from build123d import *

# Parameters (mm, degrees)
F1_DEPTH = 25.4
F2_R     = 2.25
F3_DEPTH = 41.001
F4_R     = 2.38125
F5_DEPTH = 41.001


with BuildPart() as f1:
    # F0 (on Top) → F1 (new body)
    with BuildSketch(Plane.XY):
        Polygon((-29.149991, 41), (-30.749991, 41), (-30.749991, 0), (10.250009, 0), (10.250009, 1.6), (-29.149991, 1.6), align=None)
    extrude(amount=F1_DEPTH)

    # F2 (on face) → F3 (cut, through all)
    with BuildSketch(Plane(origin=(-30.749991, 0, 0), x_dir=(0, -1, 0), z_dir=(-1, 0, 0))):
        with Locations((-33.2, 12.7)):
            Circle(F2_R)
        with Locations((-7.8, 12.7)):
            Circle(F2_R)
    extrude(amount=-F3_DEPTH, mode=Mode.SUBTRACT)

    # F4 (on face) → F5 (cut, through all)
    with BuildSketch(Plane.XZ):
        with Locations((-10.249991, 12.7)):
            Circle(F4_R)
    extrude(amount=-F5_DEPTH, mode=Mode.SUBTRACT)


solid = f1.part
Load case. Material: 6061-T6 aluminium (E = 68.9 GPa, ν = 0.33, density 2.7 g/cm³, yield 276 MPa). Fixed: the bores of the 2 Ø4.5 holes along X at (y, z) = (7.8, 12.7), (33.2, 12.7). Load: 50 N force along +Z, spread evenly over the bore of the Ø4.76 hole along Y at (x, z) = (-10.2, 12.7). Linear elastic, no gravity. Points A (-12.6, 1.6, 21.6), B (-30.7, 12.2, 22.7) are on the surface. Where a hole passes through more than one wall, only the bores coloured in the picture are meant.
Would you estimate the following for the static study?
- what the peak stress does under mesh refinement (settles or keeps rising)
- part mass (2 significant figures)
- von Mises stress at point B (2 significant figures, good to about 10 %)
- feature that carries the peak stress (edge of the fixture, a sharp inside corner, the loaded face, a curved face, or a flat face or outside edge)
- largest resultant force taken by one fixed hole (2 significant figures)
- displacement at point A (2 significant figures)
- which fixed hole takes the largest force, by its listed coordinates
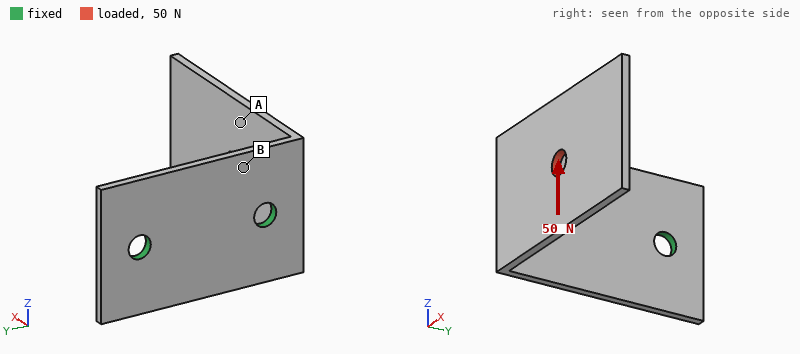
keeps rising
8.6 g
24 MPa
edge of the fixture
59 N
0.098 mm
(7.8, 12.7)
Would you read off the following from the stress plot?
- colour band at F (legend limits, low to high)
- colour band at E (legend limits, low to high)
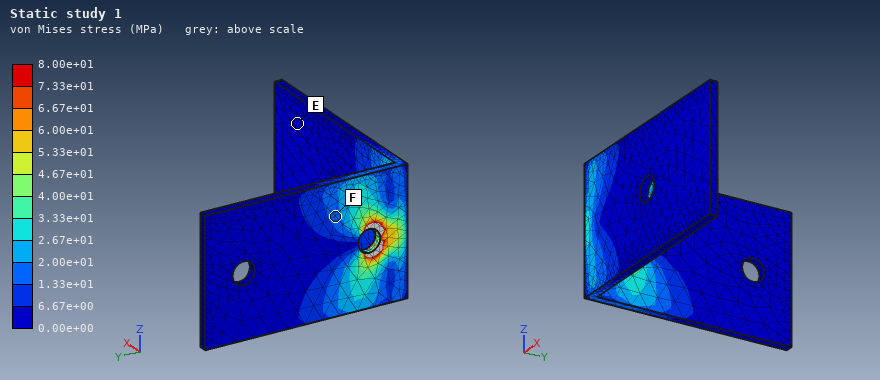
1.33e+01 to 2.00e+01 MPa
0.00e+00 to 6.67e+00 MPa
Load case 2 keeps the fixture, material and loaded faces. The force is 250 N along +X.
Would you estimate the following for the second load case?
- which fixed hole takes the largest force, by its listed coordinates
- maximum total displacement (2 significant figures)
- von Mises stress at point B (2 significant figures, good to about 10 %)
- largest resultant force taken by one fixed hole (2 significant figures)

(7.8, 12.7)
0.34 mm
17 MPa
260 N
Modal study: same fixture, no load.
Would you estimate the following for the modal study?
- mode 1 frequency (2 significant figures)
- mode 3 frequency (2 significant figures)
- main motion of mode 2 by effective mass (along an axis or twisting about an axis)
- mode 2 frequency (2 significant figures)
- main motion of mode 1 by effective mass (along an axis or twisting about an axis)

650 Hz
2700 Hz
along Z
1400 Hz
along Y
